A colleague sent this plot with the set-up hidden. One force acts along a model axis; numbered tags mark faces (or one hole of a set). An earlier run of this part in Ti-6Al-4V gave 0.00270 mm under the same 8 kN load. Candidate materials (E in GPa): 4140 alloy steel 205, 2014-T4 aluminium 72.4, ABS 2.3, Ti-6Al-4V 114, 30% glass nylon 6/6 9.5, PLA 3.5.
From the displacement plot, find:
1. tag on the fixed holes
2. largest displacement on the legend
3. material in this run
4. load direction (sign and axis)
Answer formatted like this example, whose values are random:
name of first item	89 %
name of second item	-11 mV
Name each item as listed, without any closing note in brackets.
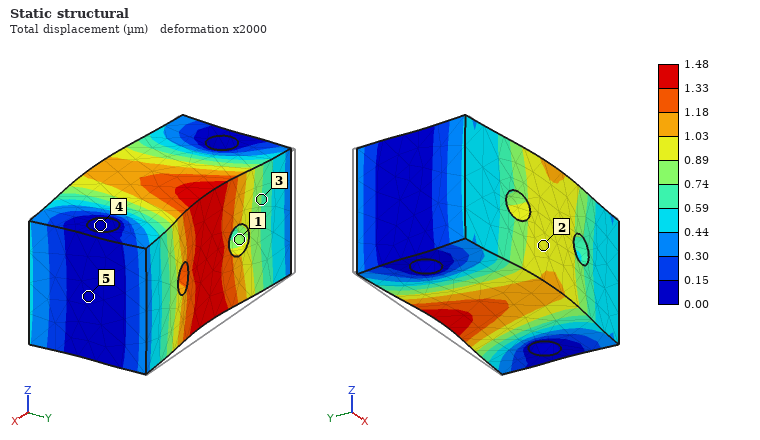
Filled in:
tag on the fixed holes	4
largest displacement on the legend	1.48 µm
material in this run	4140 alloy steel
load direction	-Y
